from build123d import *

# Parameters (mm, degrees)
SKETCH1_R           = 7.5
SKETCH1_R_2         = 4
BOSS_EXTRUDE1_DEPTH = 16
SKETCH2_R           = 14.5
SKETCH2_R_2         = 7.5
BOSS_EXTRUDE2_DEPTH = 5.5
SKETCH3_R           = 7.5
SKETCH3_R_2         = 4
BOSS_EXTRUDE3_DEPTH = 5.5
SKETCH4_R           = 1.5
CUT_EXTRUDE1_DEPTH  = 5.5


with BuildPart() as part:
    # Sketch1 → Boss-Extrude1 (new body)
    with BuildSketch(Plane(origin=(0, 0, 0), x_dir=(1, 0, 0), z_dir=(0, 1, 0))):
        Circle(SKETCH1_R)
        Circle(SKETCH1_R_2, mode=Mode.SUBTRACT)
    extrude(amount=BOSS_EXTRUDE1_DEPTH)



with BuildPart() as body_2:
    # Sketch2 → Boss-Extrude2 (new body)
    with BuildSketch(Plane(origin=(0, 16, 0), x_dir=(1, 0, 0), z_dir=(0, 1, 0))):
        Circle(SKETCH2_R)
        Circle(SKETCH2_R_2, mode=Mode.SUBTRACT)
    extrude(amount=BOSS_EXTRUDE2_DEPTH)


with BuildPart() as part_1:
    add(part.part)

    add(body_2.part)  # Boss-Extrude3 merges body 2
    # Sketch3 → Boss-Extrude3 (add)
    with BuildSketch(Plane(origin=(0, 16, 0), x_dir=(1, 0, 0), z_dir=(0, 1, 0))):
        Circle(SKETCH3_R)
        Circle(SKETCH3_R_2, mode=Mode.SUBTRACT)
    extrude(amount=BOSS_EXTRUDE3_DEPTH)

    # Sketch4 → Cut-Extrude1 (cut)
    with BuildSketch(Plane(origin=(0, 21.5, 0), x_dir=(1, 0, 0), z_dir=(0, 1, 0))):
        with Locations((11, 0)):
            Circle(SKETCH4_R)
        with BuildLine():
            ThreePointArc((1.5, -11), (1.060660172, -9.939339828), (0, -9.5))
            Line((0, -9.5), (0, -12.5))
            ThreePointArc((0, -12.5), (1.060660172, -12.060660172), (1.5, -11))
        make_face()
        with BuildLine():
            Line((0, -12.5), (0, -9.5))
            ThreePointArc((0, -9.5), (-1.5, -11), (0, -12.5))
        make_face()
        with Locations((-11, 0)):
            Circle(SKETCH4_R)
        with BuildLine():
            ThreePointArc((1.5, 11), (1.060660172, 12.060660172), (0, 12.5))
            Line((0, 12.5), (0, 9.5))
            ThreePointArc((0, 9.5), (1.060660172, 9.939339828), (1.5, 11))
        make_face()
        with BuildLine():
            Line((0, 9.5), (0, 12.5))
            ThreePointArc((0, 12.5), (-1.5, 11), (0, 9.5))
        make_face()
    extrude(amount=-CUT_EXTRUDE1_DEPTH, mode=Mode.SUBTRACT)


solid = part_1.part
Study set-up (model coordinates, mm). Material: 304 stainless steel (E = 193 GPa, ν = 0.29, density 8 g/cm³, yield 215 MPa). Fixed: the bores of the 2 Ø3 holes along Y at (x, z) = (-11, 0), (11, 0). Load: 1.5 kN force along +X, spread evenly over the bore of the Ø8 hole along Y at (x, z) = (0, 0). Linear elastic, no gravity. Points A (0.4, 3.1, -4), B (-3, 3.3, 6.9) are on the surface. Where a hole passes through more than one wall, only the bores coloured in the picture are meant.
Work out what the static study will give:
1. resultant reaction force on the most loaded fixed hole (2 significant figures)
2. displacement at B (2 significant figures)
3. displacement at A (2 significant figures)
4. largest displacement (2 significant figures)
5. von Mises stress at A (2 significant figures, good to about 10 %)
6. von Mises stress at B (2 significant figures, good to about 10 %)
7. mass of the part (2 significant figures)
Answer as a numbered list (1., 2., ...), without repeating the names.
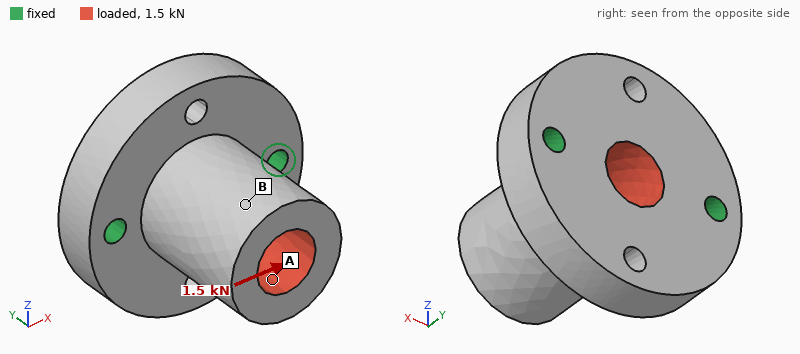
1. 980 N
2. 4.5 µm
3. 4.7 µm
4. 5.8 µm
5. 10 MPa
6. 4.8 MPa
7. 42 g
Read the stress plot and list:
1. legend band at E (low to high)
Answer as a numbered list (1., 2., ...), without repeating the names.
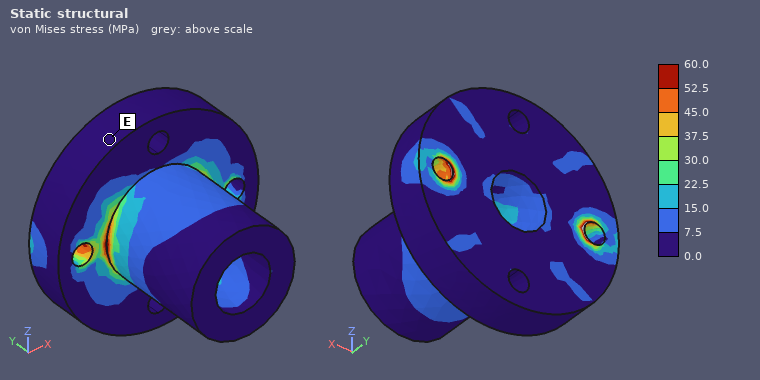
1. 0.0 to 7.5 MPa
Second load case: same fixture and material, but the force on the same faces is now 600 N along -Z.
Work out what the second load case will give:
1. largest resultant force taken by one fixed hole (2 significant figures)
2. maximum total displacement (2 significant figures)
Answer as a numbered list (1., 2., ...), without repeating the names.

1. 300 N
2. 7.2 µm
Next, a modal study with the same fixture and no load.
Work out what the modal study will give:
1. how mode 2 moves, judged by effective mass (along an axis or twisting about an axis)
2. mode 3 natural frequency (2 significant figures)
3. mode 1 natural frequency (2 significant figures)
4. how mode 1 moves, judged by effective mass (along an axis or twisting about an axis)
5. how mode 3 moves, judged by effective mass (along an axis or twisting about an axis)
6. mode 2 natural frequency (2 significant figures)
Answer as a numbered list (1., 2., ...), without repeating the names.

1. along X
2. 23 kHz
3. 10 kHz
4. along Z
5. along Y
6. 20 kHz
